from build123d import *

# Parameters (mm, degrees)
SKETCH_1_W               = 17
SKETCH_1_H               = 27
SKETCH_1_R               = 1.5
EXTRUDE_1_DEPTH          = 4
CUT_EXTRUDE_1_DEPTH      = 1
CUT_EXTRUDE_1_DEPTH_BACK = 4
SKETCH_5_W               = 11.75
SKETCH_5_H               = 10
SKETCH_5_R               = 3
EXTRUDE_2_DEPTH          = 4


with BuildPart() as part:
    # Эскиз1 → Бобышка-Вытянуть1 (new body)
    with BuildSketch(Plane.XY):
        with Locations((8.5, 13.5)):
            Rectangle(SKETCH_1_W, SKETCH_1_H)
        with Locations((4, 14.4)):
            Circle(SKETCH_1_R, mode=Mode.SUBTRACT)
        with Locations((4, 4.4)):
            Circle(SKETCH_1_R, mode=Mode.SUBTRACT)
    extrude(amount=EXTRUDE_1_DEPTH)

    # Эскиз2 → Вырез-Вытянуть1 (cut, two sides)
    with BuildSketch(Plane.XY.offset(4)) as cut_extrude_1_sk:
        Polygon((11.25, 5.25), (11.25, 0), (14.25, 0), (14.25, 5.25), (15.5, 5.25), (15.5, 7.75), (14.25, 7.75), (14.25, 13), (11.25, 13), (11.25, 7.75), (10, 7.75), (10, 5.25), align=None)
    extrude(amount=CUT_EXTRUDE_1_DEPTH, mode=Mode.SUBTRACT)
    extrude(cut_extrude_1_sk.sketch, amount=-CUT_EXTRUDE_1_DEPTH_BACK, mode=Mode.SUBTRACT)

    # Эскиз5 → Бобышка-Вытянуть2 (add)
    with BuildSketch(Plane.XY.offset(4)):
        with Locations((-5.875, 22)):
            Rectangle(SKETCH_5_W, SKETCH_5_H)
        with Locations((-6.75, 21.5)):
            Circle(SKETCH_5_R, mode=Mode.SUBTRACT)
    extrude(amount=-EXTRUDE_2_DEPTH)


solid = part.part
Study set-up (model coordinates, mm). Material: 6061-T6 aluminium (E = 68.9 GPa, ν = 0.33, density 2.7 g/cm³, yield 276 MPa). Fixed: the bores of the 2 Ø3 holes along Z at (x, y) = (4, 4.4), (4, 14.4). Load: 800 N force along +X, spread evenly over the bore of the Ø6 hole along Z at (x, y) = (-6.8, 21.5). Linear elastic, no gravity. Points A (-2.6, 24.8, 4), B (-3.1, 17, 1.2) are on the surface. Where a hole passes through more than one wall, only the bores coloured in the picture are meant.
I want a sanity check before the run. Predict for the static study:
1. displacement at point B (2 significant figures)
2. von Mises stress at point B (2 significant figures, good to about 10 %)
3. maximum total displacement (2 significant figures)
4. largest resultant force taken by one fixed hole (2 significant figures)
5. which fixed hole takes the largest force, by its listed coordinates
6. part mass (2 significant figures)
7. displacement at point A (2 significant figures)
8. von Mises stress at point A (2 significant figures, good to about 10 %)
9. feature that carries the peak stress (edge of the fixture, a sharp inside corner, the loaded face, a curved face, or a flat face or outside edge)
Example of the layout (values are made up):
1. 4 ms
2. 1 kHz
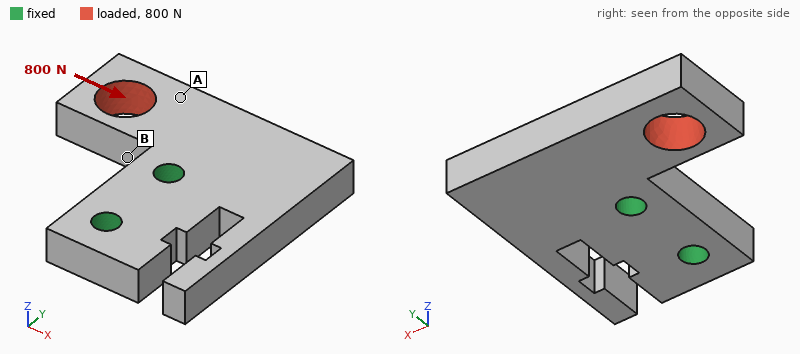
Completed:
1. 12 µm
2. 55 MPa
3. 28 µm
4. 1.1 kN
5. (4, 14.4)
6. 5.3 g
7. 20 µm
8. 24 MPa
9. edge of the fixture
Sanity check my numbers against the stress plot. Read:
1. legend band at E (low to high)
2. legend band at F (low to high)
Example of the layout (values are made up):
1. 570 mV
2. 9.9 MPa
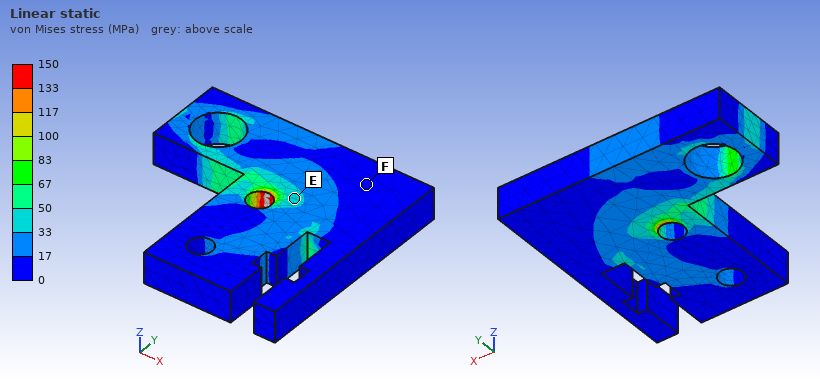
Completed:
1. 33 to 50 MPa
2. 0 to 17 MPa
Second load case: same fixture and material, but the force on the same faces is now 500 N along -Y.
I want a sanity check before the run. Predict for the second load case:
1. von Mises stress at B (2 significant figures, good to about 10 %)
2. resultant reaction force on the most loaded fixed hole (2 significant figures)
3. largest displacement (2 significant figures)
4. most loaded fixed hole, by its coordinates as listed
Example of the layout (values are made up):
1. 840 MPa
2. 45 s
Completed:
1. 65 MPa
2. 740 N
3. 61 µm
4. (4, 14.4)
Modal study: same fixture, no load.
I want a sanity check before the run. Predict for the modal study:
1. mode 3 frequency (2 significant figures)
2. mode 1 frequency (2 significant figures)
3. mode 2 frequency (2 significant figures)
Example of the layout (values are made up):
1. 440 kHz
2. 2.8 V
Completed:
1. 10 kHz
2. 8600 Hz
3. 9400 Hz
